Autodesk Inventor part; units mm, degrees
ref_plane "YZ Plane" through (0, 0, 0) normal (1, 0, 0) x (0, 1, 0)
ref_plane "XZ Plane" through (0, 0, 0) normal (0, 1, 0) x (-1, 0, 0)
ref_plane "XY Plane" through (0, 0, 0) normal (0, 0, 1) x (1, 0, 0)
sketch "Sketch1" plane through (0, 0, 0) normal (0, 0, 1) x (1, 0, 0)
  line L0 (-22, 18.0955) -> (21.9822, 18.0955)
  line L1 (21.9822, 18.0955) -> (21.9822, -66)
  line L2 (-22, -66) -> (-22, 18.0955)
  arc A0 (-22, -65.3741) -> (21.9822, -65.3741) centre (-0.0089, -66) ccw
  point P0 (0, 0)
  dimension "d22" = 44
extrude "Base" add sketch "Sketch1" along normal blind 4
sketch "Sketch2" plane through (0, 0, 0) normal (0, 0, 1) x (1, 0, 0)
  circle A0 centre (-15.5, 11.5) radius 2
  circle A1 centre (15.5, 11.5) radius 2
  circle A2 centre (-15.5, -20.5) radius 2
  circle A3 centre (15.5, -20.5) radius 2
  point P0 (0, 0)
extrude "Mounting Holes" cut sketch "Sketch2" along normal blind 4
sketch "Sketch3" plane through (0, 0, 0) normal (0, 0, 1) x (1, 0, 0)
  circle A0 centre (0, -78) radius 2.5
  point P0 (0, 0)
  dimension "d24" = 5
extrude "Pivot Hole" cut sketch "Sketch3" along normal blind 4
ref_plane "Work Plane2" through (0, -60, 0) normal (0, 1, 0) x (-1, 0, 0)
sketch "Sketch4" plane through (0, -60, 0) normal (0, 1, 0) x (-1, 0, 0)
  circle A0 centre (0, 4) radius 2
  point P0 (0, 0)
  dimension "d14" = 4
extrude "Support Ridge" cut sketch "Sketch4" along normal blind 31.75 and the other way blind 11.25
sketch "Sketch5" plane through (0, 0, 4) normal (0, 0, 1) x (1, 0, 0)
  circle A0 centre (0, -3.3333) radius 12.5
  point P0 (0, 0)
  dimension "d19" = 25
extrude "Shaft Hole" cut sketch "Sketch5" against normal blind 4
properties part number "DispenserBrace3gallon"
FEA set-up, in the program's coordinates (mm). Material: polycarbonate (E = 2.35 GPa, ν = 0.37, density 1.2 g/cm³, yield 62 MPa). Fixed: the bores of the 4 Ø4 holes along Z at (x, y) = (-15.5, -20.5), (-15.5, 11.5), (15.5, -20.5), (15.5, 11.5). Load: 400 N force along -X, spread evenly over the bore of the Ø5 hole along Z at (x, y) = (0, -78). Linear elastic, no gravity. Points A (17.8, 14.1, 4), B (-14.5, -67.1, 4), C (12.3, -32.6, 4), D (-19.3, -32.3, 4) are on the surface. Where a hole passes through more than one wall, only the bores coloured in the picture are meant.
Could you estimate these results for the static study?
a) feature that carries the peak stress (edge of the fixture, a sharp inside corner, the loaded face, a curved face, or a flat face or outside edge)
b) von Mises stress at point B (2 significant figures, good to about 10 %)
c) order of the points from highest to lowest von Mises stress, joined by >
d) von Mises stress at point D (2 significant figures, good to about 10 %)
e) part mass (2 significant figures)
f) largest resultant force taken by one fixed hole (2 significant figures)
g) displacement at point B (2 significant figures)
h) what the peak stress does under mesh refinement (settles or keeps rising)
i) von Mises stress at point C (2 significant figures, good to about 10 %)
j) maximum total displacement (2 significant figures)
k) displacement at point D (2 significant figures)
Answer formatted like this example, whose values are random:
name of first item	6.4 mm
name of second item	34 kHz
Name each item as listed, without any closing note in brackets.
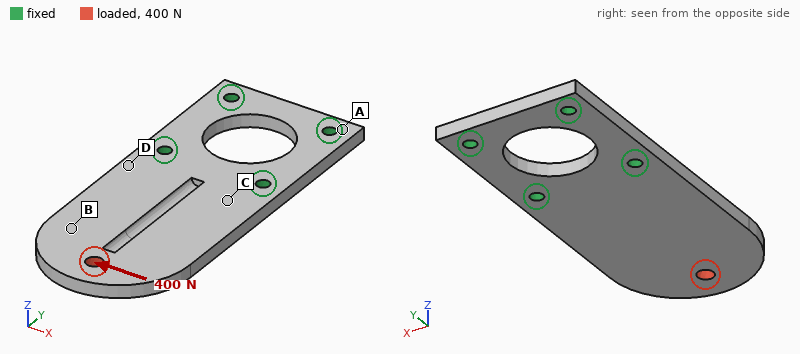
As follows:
feature that carries the peak stress	edge of the fixture
von Mises stress at point B	4.7 MPa
order of the points from highest to lowest von Mises stress, joined by >	D > C > B > A
von Mises stress at point D	12 MPa
part mass	18 g
largest resultant force taken by one fixed hole	690 N
displacement at point B	0.50 mm
what the peak stress does under mesh refinement	keeps rising
von Mises stress at point C	9.6 MPa
maximum total displacement	0.73 mm
displacement at point D	0.12 mm
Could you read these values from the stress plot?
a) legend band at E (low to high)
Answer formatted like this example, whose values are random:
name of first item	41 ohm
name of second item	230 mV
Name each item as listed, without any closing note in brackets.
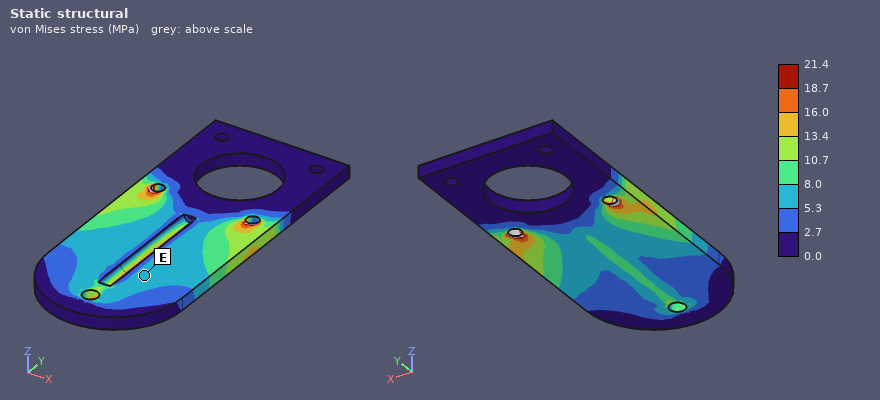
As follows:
legend band at E	5.3 to 8.0 MPa
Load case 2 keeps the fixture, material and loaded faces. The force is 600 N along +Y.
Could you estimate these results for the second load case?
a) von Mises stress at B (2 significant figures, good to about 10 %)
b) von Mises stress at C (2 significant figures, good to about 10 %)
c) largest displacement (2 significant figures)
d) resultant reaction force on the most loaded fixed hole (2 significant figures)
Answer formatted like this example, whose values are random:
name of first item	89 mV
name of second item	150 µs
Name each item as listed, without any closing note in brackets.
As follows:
von Mises stress at B	3.2 MPa
von Mises stress at C	4.3 MPa
largest displacement	0.17 mm
resultant reaction force on the most loaded fixed hole	290 N
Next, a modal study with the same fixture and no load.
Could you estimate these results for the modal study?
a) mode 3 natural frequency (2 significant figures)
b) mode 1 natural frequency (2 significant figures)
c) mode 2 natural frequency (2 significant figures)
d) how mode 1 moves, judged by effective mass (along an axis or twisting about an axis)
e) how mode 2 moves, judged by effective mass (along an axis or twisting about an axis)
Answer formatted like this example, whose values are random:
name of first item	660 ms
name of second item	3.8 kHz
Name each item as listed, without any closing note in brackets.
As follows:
mode 3 natural frequency	1300 Hz
mode 1 natural frequency	220 Hz
mode 2 natural frequency	770 Hz
how mode 1 moves, judged by effective mass	along Z
how mode 2 moves, judged by effective mass	twisting about Y
